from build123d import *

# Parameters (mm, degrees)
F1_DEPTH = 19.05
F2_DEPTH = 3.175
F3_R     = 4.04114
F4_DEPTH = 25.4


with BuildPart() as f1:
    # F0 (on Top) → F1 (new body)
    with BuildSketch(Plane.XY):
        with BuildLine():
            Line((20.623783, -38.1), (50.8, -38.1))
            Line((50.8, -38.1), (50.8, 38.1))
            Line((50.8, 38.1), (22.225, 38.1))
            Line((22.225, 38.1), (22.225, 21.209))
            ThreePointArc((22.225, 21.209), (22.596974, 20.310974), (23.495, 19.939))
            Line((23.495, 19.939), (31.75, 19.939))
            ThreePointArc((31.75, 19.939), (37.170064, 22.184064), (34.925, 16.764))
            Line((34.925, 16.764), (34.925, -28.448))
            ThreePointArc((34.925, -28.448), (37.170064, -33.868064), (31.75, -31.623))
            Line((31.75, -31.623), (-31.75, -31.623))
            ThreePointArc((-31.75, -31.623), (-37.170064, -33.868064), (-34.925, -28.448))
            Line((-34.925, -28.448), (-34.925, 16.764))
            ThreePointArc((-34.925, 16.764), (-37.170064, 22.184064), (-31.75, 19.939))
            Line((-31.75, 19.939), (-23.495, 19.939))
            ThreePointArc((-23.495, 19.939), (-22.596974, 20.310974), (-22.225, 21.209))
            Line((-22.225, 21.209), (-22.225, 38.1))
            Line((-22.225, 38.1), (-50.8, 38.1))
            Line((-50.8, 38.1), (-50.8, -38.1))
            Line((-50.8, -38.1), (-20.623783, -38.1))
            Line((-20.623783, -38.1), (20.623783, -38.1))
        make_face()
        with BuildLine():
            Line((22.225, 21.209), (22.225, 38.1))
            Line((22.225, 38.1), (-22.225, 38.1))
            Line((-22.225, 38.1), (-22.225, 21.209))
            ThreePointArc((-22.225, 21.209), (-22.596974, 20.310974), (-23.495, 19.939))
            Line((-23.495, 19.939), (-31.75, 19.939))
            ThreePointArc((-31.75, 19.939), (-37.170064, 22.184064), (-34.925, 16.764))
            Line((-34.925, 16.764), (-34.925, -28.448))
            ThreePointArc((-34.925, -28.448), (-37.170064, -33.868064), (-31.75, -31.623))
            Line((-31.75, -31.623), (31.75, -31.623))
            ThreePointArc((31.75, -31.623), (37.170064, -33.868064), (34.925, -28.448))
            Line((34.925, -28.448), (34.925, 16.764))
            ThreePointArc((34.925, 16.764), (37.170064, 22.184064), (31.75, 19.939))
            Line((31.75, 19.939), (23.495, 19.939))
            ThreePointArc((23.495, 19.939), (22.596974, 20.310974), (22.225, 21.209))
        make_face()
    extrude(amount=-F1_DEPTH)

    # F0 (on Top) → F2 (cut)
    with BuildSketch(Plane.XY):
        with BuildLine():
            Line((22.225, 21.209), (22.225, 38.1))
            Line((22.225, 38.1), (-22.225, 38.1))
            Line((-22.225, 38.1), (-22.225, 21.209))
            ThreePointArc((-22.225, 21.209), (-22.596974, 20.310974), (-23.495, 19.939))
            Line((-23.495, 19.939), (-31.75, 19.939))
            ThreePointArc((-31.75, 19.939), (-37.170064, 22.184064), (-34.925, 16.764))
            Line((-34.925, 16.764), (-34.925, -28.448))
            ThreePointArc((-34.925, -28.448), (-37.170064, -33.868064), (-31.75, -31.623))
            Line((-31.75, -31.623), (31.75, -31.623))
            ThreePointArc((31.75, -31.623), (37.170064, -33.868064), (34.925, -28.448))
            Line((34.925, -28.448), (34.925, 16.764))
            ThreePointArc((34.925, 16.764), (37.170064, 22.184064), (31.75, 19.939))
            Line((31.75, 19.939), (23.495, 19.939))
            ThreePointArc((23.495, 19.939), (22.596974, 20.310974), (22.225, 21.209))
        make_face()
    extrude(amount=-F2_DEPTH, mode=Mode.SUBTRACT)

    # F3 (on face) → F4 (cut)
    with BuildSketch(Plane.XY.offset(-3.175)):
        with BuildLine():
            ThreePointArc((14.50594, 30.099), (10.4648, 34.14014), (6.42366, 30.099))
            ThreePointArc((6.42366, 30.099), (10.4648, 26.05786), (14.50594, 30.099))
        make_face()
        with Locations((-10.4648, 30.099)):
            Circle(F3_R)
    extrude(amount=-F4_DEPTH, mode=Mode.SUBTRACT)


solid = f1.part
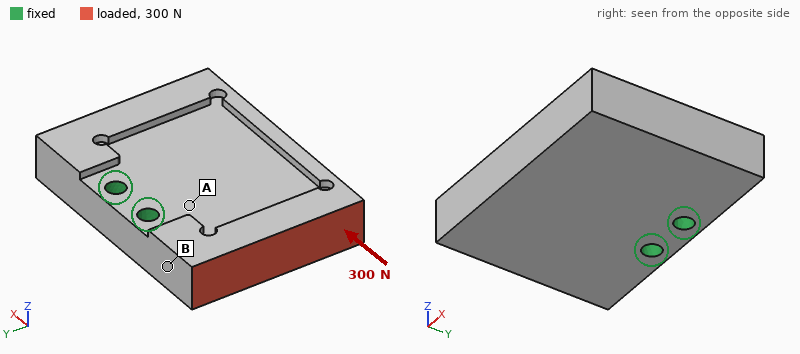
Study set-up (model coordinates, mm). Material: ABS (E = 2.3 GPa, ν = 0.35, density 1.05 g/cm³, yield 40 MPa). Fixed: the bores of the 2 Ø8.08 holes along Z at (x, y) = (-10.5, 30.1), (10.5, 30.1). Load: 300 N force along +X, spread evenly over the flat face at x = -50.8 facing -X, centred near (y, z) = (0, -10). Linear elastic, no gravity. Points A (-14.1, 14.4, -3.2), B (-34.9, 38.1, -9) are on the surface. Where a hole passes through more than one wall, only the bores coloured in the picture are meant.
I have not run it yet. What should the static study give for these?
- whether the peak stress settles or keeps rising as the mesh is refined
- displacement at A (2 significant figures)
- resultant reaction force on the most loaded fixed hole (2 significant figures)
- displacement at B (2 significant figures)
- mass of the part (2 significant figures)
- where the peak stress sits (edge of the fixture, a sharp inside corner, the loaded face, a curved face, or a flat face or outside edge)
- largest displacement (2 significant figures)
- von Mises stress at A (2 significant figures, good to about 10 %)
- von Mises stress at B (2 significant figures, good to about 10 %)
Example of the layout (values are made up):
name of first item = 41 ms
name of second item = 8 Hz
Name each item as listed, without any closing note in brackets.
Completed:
whether the peak stress settles or keeps rising as the mesh is refined = keeps rising
displacement at A = 16 µm
resultant reaction force on the most loaded fixed hole = 350 N
displacement at B = 23 µm
mass of the part = 140 g
where the peak stress sits = edge of the fixture
largest displacement = 74 µm
von Mises stress at A = 0.84 MPa
von Mises stress at B = 0.26 MPa
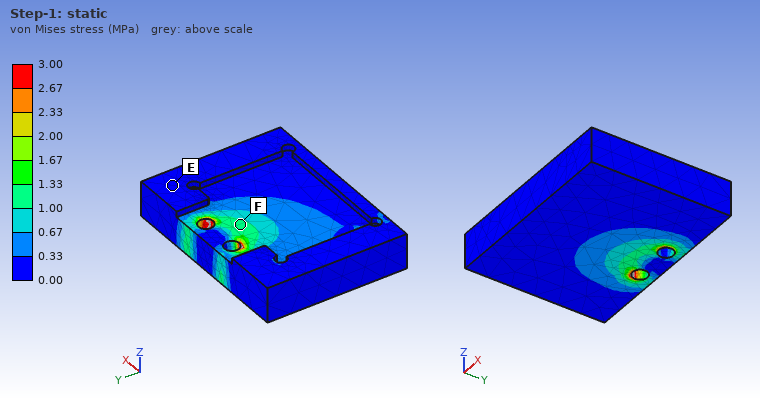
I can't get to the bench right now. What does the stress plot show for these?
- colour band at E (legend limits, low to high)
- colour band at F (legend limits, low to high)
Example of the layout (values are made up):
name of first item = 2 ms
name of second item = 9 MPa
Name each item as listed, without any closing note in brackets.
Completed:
colour band at E = 0.00 to 0.33 MPa
colour band at F = 1.00 to 1.33 MPa
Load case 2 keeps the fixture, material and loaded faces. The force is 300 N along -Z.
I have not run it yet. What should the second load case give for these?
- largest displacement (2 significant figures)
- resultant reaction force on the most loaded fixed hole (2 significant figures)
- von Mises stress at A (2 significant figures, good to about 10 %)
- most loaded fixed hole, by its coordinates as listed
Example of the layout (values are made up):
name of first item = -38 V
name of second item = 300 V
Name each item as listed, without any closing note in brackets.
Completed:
largest displacement = 0.52 mm
resultant reaction force on the most loaded fixed hole = 430 N
von Mises stress at A = 3.7 MPa
most loaded fixed hole, by its coordinates as listed = (-10.5, 30.1)
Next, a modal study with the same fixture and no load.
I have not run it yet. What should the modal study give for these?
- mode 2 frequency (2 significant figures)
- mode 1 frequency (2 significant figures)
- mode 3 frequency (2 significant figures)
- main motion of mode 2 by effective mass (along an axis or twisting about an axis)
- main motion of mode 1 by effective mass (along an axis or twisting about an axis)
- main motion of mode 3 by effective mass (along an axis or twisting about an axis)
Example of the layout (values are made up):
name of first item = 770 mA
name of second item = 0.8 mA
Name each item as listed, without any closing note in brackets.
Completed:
mode 2 frequency = 870 Hz
mode 1 frequency = 630 Hz
mode 3 frequency = 980 Hz
main motion of mode 2 by effective mass = twisting about Y
main motion of mode 1 by effective mass = along Z
main motion of mode 3 by effective mass = along X
